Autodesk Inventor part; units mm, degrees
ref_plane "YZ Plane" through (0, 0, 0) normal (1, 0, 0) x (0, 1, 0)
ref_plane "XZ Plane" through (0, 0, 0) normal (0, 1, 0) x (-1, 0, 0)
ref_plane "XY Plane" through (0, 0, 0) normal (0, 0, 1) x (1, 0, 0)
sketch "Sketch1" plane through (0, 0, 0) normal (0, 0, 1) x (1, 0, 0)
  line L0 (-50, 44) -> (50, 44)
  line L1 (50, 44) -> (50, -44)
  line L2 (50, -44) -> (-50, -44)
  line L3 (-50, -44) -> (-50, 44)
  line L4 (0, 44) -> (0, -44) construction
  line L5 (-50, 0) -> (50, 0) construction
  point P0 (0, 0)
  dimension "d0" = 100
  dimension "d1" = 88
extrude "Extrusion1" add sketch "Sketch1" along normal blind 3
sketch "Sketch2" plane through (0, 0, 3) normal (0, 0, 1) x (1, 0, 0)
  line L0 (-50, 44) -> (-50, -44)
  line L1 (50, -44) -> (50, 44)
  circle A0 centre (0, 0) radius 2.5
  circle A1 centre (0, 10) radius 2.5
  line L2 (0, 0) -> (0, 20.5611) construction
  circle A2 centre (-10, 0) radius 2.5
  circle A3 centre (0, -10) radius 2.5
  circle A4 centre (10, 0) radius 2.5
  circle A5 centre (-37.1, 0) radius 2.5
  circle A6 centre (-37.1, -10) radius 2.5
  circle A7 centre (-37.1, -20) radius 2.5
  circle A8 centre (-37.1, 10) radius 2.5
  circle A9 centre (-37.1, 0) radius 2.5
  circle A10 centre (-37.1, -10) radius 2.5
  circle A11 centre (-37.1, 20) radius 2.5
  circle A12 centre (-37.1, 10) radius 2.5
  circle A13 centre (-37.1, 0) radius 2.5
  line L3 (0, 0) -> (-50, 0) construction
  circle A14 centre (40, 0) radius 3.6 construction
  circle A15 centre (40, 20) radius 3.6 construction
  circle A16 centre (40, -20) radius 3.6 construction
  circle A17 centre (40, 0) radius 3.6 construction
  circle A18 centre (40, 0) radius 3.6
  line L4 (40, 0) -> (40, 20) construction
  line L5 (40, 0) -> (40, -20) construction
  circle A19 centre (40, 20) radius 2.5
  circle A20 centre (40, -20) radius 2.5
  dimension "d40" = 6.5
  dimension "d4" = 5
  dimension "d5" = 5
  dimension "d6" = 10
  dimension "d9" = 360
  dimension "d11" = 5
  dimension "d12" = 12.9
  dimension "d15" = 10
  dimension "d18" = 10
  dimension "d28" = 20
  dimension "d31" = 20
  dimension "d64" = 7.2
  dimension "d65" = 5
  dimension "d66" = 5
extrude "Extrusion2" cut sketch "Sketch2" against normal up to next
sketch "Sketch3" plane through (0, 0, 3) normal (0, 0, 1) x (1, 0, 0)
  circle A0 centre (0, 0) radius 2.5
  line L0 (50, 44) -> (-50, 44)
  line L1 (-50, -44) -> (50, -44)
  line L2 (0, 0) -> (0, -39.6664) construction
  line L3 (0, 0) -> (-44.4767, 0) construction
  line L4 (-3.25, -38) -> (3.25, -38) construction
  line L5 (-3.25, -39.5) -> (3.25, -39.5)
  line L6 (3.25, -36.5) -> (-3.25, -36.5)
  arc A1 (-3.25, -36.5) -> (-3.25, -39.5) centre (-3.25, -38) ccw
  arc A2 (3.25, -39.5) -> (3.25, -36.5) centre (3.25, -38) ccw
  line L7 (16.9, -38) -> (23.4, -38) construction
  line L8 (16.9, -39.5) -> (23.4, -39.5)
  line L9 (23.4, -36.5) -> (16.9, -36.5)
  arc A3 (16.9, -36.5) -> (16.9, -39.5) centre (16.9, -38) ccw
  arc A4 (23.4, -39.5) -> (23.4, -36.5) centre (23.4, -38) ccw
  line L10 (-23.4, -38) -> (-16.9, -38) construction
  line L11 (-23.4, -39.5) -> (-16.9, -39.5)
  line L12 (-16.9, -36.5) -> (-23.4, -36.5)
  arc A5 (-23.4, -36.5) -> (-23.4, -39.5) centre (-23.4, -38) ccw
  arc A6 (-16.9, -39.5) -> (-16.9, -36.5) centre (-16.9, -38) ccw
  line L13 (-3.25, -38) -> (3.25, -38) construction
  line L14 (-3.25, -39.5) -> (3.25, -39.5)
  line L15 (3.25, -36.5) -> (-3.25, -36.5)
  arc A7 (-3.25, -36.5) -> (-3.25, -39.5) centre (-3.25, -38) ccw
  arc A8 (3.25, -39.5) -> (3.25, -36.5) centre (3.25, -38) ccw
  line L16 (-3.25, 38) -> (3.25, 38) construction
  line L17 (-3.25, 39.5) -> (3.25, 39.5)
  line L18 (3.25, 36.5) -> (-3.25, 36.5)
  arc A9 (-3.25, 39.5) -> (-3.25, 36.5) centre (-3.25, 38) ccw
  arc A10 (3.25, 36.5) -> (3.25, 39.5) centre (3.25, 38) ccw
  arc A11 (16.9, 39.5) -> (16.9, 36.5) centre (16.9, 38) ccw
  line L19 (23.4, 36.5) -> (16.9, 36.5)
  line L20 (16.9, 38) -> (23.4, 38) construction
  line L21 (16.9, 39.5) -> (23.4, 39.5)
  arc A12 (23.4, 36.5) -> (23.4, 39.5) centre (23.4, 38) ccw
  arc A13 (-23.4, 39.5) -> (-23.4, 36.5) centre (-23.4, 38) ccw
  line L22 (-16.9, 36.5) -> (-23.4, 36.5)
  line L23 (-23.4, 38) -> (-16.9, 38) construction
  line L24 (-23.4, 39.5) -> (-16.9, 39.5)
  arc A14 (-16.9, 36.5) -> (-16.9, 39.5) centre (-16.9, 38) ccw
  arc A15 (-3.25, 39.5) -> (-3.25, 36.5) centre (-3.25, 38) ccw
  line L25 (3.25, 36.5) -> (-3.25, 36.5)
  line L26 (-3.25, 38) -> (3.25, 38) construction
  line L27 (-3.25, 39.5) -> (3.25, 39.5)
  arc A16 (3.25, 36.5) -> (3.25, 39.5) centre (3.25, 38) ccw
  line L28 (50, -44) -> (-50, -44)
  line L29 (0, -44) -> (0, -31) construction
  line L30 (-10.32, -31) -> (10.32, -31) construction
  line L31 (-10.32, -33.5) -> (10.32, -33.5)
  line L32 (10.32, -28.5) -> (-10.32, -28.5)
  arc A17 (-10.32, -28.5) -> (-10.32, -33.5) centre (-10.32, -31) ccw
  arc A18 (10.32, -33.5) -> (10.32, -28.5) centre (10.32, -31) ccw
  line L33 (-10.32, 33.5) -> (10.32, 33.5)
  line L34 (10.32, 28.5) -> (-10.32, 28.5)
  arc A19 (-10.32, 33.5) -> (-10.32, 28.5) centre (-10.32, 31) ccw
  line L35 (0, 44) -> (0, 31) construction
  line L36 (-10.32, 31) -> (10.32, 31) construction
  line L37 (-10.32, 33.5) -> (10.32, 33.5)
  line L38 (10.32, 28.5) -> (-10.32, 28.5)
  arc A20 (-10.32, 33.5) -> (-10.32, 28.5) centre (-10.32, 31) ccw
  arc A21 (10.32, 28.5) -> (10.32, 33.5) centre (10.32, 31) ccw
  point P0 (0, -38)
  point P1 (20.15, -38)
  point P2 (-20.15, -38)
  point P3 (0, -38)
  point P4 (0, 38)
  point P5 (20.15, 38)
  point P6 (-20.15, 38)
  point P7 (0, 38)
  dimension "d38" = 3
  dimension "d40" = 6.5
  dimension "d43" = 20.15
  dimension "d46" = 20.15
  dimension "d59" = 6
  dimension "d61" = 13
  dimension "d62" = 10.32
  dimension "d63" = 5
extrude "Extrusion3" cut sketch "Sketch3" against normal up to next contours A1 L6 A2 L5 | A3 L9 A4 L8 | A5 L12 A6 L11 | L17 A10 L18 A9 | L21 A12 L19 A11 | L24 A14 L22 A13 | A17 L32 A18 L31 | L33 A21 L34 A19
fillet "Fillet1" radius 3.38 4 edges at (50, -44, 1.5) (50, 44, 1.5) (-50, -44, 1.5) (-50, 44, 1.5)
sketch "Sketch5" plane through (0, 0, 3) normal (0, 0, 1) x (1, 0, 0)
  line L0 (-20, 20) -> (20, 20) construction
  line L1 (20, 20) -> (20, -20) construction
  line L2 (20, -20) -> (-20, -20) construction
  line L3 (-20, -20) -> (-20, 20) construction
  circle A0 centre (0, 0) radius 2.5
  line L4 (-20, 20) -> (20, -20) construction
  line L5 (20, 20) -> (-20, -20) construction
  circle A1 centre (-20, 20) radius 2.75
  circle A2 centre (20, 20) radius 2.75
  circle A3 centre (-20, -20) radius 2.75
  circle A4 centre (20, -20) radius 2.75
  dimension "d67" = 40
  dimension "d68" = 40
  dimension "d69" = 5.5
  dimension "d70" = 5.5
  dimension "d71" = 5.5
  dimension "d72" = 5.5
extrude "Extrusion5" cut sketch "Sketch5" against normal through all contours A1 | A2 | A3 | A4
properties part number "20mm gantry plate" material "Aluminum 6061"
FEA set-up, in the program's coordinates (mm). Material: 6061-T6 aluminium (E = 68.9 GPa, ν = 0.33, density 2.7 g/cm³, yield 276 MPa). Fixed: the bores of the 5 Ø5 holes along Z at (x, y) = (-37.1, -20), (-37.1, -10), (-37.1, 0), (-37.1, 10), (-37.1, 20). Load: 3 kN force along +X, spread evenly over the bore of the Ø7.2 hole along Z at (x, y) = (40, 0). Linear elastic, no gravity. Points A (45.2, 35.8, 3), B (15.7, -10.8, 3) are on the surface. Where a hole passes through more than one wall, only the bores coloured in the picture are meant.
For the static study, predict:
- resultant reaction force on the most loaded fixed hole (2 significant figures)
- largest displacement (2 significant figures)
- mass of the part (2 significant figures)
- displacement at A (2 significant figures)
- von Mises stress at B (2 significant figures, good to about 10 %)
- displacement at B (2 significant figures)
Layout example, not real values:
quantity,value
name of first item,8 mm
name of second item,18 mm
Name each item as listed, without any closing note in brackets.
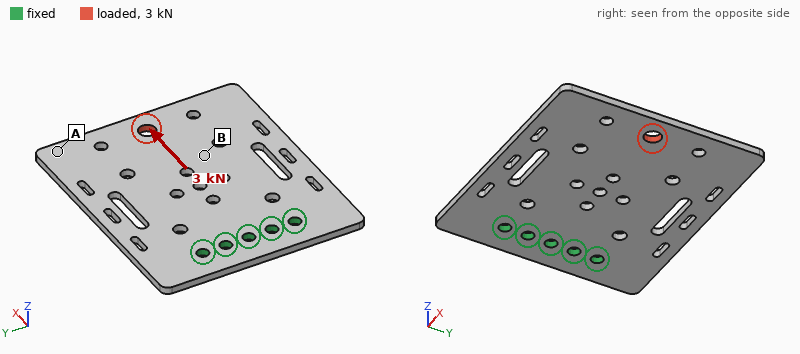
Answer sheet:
quantity,value
resultant reaction force on the most loaded fixed hole,880 N
largest displacement,34 µm
mass of the part,65 g
displacement at A,11 µm
von Mises stress at B,23 MPa
displacement at B,16 µm
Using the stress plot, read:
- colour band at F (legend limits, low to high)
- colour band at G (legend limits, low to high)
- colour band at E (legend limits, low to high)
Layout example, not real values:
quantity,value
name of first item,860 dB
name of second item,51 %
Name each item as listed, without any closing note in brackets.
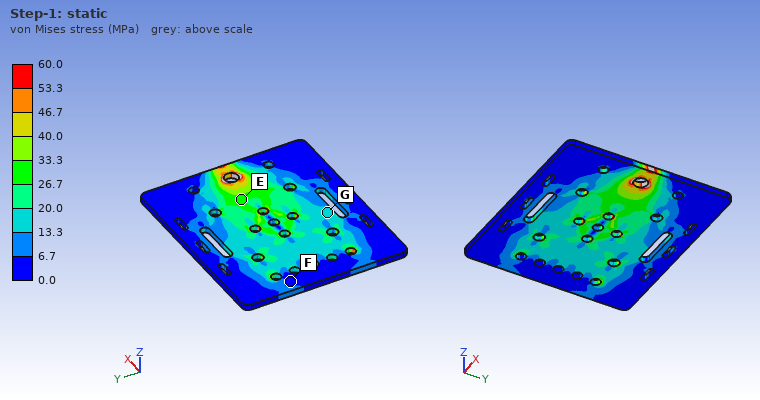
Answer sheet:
quantity,value
colour band at F,0.0 to 6.7 MPa
colour band at G,13.3 to 20.0 MPa
colour band at E,26.7 to 33.3 MPa
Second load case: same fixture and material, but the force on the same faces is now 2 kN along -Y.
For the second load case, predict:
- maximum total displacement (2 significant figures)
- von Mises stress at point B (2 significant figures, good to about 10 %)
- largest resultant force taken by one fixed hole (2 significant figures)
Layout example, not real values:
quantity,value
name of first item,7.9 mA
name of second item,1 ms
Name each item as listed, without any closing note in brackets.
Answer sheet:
quantity,value
maximum total displacement,0.14 mm
von Mises stress at point B,21 MPa
largest resultant force taken by one fixed hole,3.2 kN
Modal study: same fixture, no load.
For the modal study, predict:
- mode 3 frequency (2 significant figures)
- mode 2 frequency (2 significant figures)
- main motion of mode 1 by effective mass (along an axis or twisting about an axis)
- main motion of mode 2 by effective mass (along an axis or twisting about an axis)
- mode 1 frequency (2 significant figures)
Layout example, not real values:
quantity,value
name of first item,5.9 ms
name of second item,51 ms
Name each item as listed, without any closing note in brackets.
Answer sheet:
quantity,value
mode 3 frequency,1900 Hz
mode 2 frequency,710 Hz
main motion of mode 1 by effective mass,along Z
main motion of mode 2 by effective mass,twisting about X
mode 1 frequency,320 Hz
